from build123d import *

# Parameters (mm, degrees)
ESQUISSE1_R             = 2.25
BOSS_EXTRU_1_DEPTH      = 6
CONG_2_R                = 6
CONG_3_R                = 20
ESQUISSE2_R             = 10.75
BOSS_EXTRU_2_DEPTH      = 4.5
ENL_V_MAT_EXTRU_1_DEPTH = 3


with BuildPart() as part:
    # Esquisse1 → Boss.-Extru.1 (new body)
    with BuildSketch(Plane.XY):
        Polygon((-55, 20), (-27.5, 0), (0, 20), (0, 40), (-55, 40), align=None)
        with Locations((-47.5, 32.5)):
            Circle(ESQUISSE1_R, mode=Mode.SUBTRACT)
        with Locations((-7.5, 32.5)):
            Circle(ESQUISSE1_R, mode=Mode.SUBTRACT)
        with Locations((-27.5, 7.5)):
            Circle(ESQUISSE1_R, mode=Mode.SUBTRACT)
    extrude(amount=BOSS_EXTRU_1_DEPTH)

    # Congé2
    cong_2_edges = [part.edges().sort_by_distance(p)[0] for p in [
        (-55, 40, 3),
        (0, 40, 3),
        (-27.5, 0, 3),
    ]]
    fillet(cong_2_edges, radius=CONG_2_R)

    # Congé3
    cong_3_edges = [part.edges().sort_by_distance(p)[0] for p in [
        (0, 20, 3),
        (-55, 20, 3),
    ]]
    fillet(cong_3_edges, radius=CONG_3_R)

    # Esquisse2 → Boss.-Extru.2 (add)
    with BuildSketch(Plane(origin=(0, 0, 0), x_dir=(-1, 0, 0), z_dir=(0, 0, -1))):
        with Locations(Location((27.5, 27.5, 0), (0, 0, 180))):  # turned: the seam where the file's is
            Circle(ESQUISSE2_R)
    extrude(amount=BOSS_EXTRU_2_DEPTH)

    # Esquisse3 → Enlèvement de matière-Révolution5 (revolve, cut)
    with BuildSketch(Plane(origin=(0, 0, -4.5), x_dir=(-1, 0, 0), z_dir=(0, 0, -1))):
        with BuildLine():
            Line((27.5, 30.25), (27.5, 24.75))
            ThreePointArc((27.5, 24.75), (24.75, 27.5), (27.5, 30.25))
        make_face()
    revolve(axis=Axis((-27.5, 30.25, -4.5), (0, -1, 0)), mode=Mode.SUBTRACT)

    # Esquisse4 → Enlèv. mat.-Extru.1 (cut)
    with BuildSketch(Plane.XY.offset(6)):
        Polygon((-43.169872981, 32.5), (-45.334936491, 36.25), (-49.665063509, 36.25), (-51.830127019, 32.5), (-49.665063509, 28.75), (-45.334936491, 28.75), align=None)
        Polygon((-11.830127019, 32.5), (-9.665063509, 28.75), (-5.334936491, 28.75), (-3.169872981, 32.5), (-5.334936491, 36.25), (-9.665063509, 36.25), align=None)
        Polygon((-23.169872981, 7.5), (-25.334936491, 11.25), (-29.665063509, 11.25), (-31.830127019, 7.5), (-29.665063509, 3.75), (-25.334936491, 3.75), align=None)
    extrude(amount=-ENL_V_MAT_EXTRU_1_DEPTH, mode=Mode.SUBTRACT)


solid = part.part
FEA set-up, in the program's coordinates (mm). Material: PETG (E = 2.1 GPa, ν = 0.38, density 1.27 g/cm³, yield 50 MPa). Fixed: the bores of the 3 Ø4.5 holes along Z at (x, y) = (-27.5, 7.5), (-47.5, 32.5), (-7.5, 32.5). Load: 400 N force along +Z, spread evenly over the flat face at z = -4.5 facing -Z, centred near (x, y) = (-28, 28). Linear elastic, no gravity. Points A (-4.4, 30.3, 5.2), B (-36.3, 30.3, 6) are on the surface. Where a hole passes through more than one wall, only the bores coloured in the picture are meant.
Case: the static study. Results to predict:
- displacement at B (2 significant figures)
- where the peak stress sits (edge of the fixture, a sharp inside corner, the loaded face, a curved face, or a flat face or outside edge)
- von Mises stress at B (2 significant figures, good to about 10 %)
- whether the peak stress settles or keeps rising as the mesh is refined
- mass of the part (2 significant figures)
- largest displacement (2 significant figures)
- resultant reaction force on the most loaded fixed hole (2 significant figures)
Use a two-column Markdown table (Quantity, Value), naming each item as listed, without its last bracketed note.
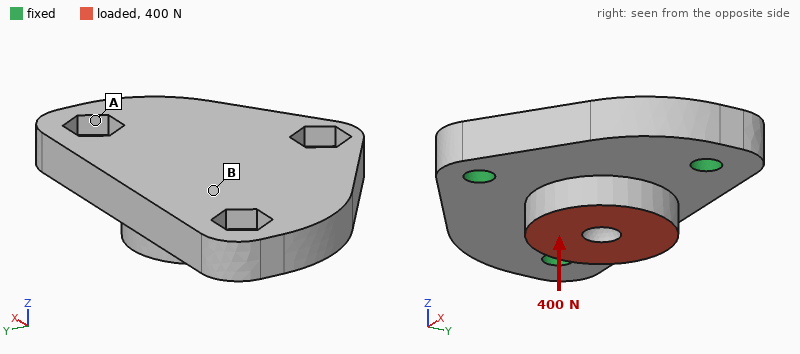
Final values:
| Quantity | Value |
|---|---|
| displacement at B | 0.096 mm |
| where the peak stress sits | edge of the fixture |
| von Mises stress at B | 6.3 MPa |
| whether the peak stress settles or keeps rising as the mesh is refined | keeps rising |
| mass of the part | 13 g |
| largest displacement | 0.16 mm |
| resultant reaction force on the most loaded fixed hole | 170 N |
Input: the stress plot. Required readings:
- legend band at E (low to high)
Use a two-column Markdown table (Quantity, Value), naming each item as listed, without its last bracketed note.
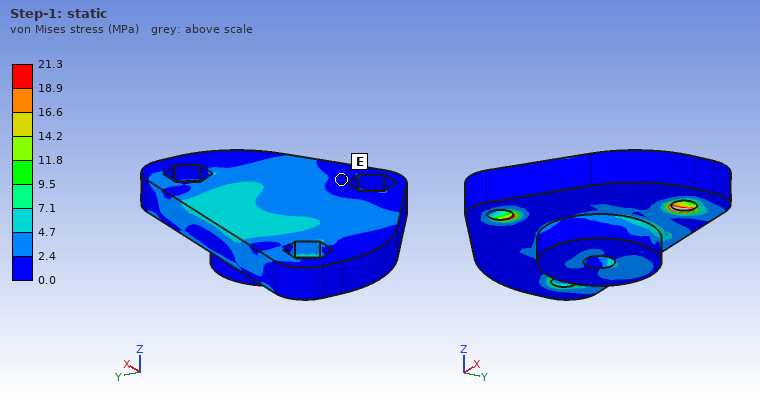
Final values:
| Quantity | Value |
|---|---|
| legend band at E | 0.0 to 2.4 MPa |
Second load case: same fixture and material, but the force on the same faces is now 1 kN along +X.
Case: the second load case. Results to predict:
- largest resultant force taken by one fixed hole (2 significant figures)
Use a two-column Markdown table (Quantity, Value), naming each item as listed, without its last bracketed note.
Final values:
| Quantity | Value |
|---|---|
| largest resultant force taken by one fixed hole | 400 N |
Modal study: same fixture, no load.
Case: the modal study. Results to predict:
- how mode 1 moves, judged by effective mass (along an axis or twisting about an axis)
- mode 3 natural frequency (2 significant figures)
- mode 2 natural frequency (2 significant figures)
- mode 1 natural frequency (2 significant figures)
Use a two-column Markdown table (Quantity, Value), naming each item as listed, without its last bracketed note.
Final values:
| Quantity | Value |
|---|---|
| how mode 1 moves, judged by effective mass | along Z |
| mode 3 natural frequency | 4600 Hz |
| mode 2 natural frequency | 4600 Hz |
| mode 1 natural frequency | 3600 Hz |
